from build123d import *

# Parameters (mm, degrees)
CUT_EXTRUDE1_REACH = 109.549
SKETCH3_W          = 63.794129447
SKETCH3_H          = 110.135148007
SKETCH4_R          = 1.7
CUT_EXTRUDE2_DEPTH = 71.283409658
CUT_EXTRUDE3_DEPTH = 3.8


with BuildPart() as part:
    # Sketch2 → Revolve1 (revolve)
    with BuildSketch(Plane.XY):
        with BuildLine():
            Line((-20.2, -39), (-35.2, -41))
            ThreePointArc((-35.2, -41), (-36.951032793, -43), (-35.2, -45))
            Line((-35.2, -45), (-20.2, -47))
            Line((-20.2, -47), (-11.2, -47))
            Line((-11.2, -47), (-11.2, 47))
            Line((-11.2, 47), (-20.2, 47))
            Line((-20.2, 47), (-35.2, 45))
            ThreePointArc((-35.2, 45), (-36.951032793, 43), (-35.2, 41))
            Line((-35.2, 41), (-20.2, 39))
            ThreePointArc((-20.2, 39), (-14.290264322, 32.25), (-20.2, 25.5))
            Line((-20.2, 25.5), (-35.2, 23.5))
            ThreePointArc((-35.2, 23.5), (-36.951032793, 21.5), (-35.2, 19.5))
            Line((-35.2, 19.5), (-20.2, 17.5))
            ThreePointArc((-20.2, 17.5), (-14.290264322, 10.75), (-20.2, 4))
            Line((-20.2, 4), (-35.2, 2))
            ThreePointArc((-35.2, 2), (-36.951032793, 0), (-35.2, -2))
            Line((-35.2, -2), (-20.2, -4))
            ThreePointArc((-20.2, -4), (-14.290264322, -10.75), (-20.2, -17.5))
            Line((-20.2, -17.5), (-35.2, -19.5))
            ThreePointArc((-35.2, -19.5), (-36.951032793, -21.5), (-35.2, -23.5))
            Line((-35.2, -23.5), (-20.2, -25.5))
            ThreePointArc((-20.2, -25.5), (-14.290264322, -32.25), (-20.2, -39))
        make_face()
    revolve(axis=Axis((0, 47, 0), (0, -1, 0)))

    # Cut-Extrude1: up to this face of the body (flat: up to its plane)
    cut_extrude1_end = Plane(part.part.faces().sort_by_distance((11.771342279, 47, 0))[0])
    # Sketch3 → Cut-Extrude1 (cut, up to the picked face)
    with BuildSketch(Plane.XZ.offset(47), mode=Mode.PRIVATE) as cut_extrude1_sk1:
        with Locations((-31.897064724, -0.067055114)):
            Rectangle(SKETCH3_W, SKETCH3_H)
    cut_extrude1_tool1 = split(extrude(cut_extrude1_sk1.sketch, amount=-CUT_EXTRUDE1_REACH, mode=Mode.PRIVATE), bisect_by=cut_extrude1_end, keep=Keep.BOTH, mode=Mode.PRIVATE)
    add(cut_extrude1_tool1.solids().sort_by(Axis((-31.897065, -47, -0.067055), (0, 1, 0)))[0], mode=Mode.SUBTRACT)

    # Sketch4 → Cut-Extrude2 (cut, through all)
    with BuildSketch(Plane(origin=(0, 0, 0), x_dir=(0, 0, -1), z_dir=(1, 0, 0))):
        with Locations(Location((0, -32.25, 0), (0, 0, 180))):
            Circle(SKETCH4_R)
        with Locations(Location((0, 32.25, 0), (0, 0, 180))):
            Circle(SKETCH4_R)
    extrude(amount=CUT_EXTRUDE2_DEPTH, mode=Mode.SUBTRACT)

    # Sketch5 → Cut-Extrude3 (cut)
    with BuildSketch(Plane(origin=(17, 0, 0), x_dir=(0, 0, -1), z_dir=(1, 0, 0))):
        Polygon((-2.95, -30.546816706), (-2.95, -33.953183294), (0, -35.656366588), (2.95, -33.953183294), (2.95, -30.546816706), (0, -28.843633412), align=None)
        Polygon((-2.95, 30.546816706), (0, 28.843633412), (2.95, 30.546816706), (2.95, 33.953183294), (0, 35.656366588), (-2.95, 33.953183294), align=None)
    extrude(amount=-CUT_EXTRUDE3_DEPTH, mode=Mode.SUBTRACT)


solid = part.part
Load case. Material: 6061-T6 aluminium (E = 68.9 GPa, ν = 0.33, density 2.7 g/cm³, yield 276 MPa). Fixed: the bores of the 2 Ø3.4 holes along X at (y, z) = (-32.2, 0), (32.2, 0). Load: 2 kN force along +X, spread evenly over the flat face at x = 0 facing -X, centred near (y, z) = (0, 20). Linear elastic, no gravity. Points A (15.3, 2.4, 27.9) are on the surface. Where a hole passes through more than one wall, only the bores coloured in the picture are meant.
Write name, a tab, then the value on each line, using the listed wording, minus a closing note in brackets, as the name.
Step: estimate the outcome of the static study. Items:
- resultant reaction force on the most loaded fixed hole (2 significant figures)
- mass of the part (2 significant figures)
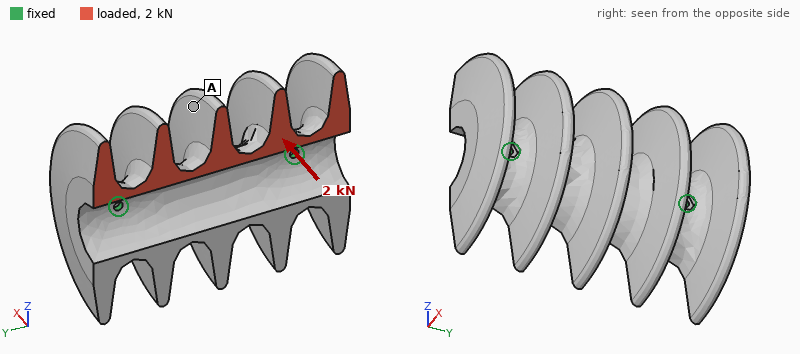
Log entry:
resultant reaction force on the most loaded fixed hole	1.0 kN
mass of the part	190 g
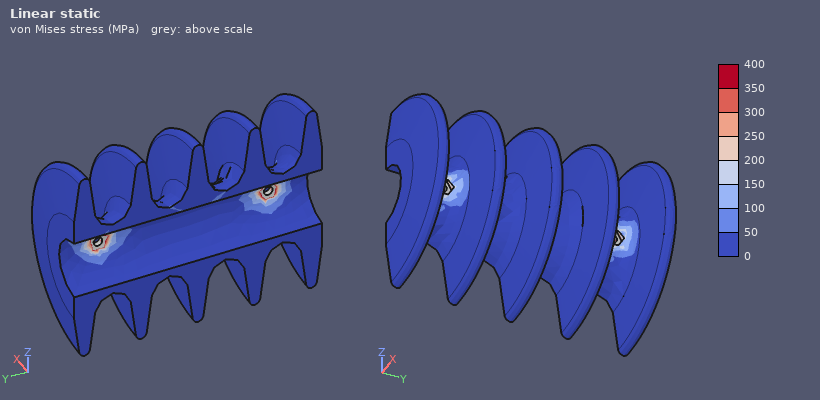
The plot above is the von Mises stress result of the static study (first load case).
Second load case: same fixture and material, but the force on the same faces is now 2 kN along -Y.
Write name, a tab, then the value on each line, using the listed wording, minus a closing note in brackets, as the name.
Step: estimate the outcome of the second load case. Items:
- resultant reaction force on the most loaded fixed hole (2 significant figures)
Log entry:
resultant reaction force on the most loaded fixed hole	1.2 kN
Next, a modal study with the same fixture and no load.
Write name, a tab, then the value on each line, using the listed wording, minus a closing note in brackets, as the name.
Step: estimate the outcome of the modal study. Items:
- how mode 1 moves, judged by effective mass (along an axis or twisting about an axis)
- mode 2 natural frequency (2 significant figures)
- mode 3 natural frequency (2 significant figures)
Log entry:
how mode 1 moves, judged by effective mass	twisting about Y
mode 2 natural frequency	1900 Hz
mode 3 natural frequency	3100 Hz
